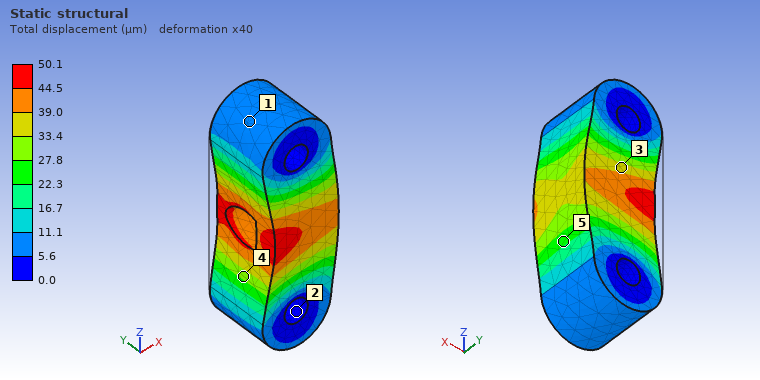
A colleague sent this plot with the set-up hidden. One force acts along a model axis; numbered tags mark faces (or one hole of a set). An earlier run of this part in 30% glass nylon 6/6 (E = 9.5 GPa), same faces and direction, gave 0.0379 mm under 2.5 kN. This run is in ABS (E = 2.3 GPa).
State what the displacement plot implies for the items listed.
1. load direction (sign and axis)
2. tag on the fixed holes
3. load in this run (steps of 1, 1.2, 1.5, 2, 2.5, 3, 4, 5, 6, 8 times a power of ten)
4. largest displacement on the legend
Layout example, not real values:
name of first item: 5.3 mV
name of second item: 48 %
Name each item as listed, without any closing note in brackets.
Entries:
load direction: +X
tag on the fixed holes: 2
load in this run: 800 N
largest displacement on the legend: 50.1 µm
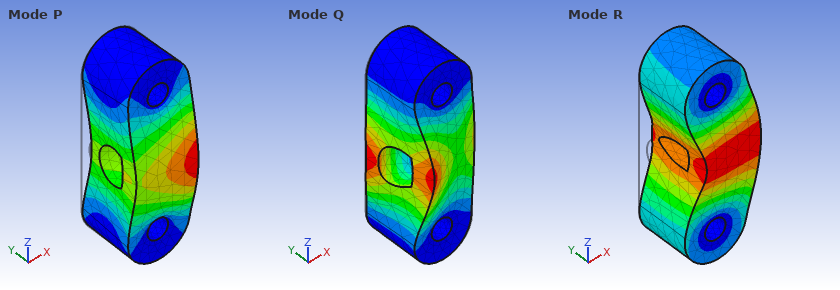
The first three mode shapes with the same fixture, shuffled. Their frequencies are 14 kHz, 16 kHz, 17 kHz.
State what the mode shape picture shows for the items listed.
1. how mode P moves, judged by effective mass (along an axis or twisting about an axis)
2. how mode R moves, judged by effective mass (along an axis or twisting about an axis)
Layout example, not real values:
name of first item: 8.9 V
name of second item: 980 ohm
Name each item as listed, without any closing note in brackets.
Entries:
how mode P moves, judged by effective mass: along Y
how mode R moves, judged by effective mass: along X
